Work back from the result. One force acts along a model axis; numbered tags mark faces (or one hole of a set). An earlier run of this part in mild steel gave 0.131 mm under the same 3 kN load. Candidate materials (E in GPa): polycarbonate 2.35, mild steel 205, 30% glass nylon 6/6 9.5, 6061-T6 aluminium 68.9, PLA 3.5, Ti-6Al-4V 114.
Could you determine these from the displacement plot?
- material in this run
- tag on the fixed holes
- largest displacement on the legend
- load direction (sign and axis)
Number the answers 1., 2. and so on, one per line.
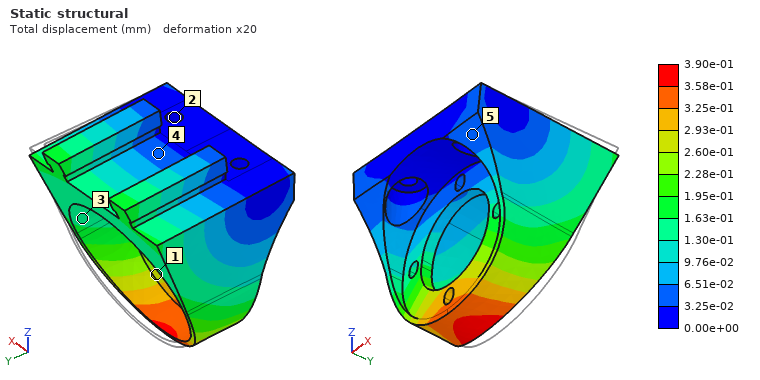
1. 6061-T6 aluminium
2. 2
3. 3.90e-01 mm
4. -Y
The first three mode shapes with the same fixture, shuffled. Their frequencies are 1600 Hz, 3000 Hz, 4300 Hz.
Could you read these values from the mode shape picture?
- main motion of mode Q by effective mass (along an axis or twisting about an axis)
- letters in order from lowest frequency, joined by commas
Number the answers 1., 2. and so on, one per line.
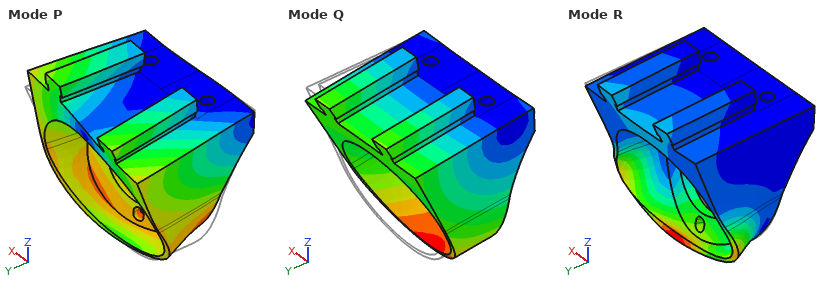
1. along Z
2. Q, P, R
